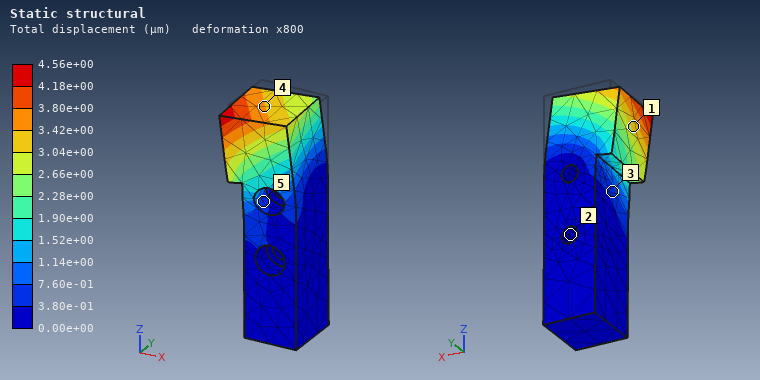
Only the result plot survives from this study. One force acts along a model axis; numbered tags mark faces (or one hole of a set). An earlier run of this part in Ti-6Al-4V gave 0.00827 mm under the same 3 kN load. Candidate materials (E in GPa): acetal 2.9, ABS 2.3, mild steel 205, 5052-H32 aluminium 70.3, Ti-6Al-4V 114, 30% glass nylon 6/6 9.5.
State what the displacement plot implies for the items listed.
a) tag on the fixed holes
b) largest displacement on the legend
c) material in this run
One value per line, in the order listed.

2
4.56e+00 µm
mild steel
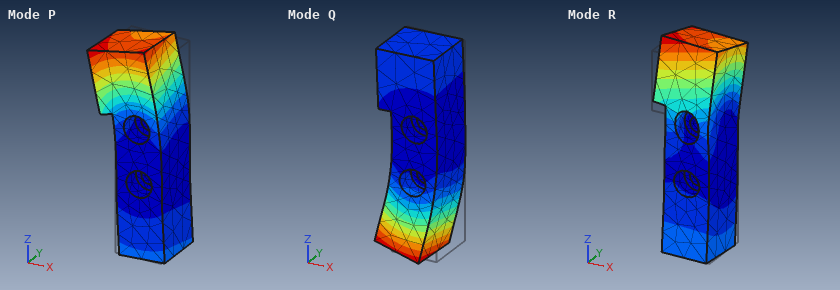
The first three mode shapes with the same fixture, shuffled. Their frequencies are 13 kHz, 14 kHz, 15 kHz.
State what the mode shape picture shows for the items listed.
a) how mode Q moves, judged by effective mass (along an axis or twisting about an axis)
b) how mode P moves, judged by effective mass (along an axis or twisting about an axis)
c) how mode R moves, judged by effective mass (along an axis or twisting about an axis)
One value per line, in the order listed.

along X
along X
along Y
